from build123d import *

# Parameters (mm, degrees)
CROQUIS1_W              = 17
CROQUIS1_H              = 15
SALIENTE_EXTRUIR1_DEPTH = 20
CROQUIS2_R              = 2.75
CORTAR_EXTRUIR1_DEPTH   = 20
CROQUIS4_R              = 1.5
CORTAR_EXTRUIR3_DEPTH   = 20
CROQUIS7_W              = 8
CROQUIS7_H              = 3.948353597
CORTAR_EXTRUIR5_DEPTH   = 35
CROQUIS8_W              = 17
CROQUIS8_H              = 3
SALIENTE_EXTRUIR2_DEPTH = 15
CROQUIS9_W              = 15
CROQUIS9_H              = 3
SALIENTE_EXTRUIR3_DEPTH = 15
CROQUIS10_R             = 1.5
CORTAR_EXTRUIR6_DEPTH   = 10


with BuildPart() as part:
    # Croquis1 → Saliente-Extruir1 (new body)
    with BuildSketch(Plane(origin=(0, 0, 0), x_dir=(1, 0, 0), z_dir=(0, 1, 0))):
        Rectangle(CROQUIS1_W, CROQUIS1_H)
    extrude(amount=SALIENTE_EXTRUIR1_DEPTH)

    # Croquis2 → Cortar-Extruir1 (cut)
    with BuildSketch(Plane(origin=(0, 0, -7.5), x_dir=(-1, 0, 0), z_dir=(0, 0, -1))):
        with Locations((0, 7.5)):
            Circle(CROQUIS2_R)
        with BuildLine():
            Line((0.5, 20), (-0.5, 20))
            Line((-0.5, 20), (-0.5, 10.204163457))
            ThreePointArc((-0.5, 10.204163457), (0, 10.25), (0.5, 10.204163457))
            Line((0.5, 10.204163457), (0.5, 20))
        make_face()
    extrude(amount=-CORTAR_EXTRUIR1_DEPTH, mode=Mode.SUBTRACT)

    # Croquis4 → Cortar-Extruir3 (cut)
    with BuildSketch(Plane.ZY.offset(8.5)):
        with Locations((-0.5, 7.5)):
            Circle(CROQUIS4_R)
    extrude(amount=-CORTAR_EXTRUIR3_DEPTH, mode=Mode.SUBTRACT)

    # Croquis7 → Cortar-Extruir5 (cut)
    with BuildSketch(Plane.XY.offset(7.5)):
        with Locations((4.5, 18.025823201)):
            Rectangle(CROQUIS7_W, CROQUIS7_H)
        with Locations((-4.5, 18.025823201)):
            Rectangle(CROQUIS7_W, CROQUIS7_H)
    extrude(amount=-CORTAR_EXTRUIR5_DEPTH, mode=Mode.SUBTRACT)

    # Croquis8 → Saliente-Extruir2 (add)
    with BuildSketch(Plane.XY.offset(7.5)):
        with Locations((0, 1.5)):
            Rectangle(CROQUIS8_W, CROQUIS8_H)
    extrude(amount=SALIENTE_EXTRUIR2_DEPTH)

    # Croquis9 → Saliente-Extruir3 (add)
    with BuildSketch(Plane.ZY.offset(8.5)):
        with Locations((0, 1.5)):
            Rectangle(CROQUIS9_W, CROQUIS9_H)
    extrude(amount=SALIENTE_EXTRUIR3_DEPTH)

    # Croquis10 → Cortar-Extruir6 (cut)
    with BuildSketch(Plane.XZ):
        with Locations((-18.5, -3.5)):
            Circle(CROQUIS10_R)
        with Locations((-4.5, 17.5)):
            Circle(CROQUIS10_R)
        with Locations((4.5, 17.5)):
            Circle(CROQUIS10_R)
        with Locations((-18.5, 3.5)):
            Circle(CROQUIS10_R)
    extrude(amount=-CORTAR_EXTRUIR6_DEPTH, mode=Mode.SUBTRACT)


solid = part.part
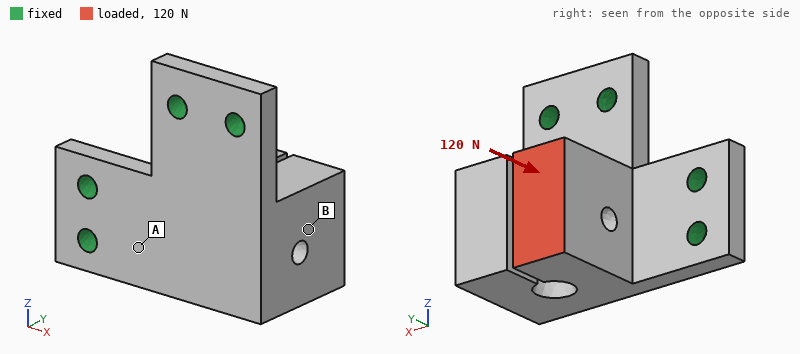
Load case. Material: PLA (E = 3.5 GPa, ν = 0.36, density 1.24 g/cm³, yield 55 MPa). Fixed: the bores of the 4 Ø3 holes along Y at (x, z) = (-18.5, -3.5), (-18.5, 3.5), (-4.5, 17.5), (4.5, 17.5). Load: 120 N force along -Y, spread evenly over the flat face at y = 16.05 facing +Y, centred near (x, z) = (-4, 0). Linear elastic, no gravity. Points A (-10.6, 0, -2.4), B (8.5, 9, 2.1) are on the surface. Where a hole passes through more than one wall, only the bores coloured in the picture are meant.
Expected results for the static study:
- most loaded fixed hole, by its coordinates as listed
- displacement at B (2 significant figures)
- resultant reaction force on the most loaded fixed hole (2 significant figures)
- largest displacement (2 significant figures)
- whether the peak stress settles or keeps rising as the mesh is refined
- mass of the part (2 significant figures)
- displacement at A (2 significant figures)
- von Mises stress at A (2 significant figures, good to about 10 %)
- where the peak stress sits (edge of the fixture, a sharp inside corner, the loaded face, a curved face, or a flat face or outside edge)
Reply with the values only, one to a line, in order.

(-18.5, -3.5)
0.27 mm
72 N
0.46 mm
keeps rising
6.1 g
0.10 mm
7.9 MPa
edge of the fixture
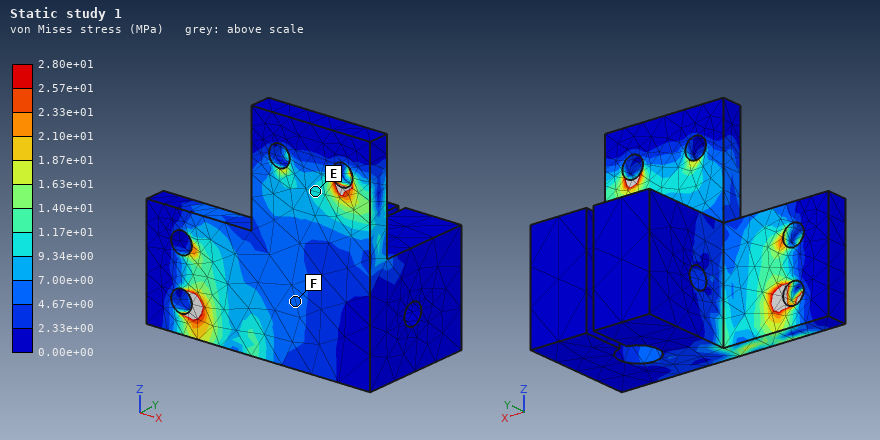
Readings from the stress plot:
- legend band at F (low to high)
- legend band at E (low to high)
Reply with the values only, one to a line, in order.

4.67e+00 to 7.00e+00 MPa
9.34e+00 to 1.17e+01 MPa
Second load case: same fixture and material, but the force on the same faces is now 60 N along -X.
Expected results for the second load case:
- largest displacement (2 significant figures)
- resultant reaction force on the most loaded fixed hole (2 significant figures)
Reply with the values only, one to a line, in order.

0.36 mm
52 N
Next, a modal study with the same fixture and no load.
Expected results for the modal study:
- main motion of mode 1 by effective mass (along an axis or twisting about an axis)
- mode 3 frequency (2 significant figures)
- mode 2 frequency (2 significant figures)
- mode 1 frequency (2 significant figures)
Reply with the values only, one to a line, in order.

along Y
4200 Hz
3100 Hz
1200 Hz
